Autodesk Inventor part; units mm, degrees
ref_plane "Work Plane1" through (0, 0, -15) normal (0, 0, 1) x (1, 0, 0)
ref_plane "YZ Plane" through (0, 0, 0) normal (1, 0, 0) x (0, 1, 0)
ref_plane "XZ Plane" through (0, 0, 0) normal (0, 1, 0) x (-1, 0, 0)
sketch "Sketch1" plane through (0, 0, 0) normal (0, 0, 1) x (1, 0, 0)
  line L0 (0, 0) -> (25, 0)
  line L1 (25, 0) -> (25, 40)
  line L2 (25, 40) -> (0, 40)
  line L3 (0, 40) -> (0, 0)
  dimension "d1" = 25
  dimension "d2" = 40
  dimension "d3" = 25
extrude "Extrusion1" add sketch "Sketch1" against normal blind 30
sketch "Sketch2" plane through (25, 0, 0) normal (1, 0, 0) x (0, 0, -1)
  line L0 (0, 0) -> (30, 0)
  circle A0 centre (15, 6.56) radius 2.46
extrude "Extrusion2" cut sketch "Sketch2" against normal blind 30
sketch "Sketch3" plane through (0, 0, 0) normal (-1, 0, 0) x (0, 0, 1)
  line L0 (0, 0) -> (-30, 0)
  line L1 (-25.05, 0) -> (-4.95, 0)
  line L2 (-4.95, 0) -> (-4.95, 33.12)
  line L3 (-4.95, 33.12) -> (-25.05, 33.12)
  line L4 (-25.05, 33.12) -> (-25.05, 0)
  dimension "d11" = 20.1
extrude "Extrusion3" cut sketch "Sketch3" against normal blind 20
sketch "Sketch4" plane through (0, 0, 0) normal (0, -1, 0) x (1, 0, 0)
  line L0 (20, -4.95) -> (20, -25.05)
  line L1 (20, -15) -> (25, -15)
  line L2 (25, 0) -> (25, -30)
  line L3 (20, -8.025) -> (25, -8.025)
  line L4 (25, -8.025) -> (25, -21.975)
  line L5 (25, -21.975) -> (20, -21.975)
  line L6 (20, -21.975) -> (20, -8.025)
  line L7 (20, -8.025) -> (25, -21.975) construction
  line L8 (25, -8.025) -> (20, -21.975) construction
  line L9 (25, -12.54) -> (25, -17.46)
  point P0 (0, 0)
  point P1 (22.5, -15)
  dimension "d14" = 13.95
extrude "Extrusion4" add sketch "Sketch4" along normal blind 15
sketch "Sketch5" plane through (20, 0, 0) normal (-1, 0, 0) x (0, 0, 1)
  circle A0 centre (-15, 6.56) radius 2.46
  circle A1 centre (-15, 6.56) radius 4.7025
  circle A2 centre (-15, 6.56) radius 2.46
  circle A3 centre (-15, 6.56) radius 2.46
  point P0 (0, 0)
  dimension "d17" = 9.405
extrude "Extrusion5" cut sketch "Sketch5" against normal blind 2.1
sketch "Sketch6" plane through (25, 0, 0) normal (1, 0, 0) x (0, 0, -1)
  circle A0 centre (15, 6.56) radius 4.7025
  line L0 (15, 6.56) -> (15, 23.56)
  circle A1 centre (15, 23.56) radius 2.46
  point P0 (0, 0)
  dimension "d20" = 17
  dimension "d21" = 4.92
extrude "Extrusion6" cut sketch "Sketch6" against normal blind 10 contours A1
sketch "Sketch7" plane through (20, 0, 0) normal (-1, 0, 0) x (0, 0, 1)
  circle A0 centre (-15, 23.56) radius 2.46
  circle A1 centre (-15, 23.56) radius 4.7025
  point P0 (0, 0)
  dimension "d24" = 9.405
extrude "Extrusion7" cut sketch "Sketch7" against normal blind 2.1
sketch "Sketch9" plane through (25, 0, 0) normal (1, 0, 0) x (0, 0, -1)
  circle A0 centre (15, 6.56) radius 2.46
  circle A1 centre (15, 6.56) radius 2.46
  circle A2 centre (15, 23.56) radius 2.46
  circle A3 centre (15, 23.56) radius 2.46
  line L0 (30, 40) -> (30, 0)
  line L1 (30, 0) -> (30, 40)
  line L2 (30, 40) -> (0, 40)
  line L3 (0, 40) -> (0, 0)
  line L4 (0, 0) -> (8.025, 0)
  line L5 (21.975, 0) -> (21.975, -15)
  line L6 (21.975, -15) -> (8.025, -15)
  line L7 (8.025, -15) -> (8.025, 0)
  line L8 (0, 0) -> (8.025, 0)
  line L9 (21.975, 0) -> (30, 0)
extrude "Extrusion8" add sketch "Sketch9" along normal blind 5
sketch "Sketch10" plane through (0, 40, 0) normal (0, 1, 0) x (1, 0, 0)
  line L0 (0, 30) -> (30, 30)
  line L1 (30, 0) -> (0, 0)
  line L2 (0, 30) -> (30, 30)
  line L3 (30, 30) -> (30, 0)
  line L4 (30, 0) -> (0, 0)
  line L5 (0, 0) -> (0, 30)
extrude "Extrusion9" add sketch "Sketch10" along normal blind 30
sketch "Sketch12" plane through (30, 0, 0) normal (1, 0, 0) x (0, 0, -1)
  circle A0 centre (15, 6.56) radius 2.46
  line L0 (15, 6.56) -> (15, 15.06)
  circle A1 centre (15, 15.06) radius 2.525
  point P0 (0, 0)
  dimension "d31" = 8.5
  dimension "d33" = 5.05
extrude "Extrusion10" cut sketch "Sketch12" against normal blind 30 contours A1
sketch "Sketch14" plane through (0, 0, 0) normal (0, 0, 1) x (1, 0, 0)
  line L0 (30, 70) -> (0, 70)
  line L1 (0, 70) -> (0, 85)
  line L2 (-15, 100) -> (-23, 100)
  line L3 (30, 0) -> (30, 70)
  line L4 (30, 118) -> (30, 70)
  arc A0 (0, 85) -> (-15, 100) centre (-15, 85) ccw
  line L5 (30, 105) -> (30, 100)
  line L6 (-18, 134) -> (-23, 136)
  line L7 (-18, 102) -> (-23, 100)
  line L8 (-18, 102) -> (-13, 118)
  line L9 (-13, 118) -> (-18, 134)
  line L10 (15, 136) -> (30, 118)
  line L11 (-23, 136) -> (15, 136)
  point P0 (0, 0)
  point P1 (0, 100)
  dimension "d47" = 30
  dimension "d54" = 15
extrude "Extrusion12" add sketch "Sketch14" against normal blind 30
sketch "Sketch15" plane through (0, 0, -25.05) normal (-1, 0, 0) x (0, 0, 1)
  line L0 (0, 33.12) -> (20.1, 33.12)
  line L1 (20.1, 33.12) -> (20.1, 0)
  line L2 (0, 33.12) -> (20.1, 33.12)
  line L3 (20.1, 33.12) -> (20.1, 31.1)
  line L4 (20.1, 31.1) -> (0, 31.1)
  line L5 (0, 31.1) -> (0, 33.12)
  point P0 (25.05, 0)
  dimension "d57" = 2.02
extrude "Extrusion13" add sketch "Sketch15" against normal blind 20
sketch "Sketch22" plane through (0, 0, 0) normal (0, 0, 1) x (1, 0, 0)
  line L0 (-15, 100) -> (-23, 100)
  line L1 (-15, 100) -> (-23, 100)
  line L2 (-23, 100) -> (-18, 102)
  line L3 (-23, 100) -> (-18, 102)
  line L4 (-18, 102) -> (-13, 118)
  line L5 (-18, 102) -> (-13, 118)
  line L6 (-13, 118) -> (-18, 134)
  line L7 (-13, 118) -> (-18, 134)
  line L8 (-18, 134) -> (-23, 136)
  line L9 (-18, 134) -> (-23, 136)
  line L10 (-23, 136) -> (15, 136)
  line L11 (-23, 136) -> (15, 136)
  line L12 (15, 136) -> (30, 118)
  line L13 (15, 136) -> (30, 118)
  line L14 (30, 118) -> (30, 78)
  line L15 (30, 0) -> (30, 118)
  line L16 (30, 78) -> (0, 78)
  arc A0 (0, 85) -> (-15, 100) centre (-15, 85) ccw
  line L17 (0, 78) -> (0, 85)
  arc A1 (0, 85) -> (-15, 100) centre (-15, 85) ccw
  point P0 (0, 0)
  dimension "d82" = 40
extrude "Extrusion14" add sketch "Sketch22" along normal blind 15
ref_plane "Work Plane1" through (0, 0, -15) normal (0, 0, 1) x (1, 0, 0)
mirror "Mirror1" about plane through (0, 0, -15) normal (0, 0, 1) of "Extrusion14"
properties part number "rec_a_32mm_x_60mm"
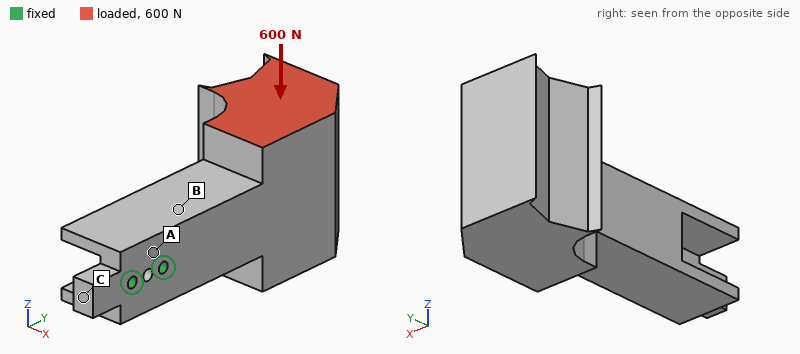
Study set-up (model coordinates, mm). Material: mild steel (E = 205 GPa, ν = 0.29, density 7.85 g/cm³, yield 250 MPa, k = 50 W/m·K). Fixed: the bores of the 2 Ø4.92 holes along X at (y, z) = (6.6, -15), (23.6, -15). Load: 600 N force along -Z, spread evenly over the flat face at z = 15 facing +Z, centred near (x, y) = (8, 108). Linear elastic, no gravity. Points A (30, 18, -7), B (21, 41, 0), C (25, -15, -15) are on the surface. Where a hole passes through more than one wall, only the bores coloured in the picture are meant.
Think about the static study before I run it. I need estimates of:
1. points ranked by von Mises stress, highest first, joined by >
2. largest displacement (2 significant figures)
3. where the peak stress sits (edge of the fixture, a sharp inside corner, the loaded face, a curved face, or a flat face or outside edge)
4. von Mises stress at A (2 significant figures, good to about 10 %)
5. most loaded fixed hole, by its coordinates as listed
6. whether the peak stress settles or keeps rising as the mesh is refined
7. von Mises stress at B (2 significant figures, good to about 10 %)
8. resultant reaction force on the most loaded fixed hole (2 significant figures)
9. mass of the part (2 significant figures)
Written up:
A > B > C
45 µm
edge of the fixture
18 MPa
(23.6, -15)
keeps rising
11 MPa
2.8 kN
1.5 kg
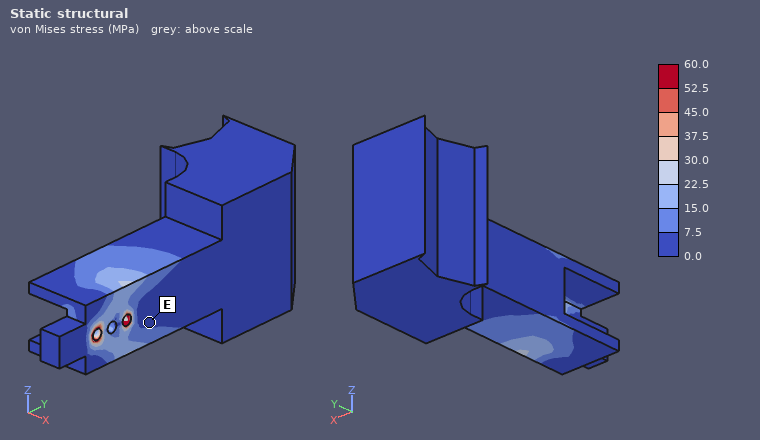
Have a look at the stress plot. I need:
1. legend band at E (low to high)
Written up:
0.0 to 7.5 MPa
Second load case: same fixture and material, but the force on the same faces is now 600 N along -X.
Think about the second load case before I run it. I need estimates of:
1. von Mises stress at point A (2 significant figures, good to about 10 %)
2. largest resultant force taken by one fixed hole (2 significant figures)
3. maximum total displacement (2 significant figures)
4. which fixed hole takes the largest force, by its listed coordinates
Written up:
22 MPa
2.6 kN
71 µm
(23.6, -15)
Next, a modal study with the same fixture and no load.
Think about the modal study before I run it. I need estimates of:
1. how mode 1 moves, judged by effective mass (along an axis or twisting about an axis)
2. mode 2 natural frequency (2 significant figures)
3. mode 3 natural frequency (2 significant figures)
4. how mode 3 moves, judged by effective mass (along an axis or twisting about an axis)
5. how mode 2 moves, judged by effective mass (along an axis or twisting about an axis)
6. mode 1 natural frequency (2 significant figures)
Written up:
along X
650 Hz
1500 Hz
twisting about Y
along Z
570 Hz
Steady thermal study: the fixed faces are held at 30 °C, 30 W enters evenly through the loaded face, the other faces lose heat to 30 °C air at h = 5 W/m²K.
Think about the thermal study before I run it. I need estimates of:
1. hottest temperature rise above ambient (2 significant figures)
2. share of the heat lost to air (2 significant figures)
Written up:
62 K
17 %
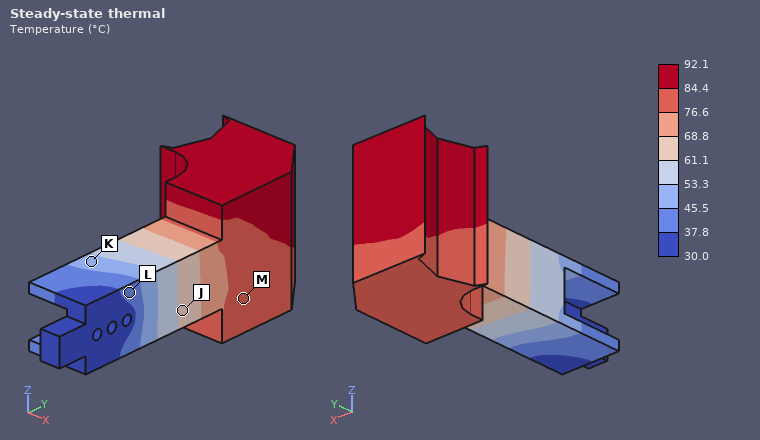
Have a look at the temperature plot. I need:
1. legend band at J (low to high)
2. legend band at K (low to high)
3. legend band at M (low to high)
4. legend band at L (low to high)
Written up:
61.1 to 68.8 °C
45.5 to 53.3 °C
76.6 to 84.4 °C
37.8 to 45.5 °C
